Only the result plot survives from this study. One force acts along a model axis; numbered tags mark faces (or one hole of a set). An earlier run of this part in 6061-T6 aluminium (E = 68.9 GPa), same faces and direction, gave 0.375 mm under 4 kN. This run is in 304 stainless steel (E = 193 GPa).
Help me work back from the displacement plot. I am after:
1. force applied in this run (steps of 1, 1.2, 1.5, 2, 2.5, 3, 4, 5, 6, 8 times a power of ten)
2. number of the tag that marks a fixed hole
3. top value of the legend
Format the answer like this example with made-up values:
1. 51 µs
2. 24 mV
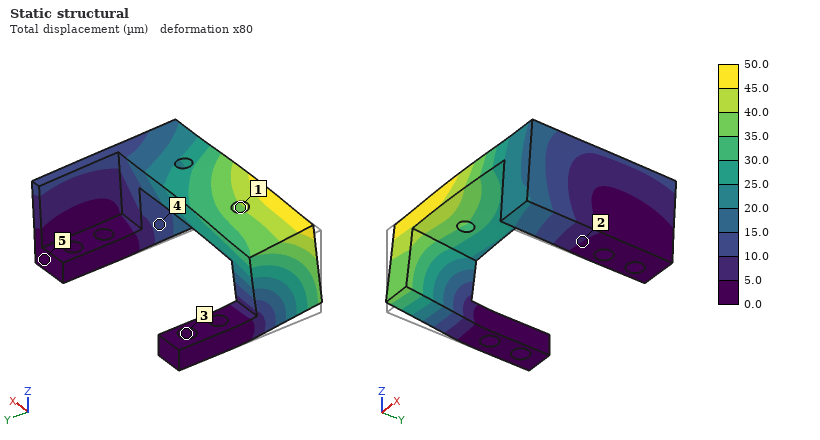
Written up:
1. 1.5 kN
2. 3
3. 50.0 µm
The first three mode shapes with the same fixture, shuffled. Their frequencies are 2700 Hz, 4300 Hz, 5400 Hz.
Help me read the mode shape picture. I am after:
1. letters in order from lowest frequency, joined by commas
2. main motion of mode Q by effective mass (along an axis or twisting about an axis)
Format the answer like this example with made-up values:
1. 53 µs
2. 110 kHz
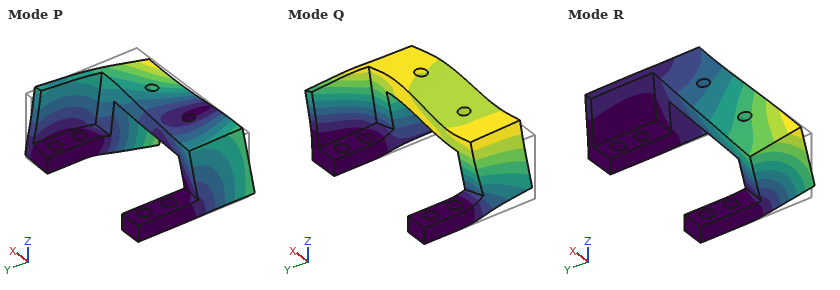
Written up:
1. R, Q, P
2. along X
